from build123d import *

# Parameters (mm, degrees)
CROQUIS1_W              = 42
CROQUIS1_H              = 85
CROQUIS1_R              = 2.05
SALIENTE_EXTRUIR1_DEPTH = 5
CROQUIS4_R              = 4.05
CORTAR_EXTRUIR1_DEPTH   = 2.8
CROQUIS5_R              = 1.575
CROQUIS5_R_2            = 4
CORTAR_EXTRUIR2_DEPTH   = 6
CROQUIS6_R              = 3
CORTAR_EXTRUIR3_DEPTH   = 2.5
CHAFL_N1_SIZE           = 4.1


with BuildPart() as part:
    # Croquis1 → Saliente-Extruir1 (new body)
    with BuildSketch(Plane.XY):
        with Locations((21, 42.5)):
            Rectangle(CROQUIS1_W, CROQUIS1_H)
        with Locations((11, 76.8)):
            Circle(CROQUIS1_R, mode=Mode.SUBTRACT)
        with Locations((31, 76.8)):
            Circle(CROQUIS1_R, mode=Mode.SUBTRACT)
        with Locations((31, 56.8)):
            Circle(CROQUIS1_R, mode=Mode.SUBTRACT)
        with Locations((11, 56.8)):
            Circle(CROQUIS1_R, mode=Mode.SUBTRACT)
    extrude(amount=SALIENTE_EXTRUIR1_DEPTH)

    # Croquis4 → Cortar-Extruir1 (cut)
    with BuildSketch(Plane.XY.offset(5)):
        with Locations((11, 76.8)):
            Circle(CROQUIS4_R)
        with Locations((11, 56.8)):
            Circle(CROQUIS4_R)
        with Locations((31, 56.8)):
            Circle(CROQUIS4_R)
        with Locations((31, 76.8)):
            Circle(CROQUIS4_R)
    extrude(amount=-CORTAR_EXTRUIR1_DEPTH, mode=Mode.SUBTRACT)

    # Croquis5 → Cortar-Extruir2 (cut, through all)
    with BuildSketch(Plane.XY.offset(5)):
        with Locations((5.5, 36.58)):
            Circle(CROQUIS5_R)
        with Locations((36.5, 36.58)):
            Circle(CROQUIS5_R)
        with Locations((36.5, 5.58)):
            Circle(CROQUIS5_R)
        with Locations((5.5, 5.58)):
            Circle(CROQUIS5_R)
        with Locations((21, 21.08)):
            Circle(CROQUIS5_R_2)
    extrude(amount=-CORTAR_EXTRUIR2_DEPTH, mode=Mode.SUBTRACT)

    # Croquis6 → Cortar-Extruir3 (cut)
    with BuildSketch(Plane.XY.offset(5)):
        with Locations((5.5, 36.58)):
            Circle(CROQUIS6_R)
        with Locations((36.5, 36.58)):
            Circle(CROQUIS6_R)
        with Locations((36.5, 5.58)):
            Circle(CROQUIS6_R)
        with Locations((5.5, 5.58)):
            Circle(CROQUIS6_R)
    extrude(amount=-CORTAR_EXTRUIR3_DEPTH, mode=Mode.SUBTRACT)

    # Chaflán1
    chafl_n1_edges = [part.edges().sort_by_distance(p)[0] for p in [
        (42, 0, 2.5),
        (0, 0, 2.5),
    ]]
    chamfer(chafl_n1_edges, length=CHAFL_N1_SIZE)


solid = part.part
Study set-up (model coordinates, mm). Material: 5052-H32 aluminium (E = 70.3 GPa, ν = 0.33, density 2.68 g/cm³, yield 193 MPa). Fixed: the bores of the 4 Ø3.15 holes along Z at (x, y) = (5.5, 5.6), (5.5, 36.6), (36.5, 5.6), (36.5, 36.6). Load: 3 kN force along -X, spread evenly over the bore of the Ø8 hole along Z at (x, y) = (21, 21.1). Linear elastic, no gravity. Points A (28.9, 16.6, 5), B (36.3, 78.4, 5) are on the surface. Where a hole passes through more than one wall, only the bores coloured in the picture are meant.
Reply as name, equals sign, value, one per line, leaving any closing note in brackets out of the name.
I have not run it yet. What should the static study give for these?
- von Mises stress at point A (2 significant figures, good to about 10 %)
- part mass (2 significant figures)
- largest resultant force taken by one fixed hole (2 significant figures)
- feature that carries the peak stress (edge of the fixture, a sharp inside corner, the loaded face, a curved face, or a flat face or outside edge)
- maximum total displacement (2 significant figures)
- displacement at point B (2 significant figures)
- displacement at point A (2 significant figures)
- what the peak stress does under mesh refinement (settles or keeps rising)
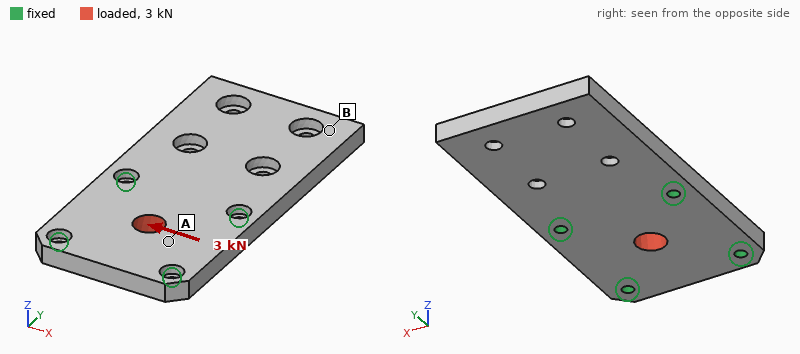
von Mises stress at point A = 16 MPa
part mass = 44 g
largest resultant force taken by one fixed hole = 810 N
feature that carries the peak stress = edge of the fixture
maximum total displacement = 7.2 µm
displacement at point B = 1.5 µm
displacement at point A = 5.2 µm
what the peak stress does under mesh refinement = keeps rising
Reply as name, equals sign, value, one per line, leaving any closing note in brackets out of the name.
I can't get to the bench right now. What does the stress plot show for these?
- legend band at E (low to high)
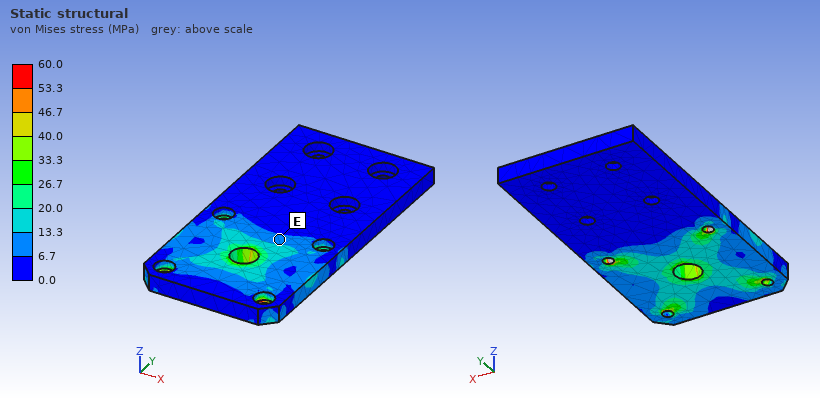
legend band at E = 6.7 to 13.3 MPa
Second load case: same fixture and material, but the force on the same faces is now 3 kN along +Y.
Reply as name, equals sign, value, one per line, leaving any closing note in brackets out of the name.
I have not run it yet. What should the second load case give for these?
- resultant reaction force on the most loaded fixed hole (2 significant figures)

resultant reaction force on the most loaded fixed hole = 840 N
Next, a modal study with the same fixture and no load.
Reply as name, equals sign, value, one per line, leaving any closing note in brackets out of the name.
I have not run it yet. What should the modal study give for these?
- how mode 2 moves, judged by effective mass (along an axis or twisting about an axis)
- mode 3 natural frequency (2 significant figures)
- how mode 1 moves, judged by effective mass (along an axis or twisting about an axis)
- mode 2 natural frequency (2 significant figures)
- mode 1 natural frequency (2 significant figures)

how mode 2 moves, judged by effective mass = twisting about Y
mode 3 natural frequency = 8800 Hz
how mode 1 moves, judged by effective mass = along Z
mode 2 natural frequency = 4200 Hz
mode 1 natural frequency = 1500 Hz
